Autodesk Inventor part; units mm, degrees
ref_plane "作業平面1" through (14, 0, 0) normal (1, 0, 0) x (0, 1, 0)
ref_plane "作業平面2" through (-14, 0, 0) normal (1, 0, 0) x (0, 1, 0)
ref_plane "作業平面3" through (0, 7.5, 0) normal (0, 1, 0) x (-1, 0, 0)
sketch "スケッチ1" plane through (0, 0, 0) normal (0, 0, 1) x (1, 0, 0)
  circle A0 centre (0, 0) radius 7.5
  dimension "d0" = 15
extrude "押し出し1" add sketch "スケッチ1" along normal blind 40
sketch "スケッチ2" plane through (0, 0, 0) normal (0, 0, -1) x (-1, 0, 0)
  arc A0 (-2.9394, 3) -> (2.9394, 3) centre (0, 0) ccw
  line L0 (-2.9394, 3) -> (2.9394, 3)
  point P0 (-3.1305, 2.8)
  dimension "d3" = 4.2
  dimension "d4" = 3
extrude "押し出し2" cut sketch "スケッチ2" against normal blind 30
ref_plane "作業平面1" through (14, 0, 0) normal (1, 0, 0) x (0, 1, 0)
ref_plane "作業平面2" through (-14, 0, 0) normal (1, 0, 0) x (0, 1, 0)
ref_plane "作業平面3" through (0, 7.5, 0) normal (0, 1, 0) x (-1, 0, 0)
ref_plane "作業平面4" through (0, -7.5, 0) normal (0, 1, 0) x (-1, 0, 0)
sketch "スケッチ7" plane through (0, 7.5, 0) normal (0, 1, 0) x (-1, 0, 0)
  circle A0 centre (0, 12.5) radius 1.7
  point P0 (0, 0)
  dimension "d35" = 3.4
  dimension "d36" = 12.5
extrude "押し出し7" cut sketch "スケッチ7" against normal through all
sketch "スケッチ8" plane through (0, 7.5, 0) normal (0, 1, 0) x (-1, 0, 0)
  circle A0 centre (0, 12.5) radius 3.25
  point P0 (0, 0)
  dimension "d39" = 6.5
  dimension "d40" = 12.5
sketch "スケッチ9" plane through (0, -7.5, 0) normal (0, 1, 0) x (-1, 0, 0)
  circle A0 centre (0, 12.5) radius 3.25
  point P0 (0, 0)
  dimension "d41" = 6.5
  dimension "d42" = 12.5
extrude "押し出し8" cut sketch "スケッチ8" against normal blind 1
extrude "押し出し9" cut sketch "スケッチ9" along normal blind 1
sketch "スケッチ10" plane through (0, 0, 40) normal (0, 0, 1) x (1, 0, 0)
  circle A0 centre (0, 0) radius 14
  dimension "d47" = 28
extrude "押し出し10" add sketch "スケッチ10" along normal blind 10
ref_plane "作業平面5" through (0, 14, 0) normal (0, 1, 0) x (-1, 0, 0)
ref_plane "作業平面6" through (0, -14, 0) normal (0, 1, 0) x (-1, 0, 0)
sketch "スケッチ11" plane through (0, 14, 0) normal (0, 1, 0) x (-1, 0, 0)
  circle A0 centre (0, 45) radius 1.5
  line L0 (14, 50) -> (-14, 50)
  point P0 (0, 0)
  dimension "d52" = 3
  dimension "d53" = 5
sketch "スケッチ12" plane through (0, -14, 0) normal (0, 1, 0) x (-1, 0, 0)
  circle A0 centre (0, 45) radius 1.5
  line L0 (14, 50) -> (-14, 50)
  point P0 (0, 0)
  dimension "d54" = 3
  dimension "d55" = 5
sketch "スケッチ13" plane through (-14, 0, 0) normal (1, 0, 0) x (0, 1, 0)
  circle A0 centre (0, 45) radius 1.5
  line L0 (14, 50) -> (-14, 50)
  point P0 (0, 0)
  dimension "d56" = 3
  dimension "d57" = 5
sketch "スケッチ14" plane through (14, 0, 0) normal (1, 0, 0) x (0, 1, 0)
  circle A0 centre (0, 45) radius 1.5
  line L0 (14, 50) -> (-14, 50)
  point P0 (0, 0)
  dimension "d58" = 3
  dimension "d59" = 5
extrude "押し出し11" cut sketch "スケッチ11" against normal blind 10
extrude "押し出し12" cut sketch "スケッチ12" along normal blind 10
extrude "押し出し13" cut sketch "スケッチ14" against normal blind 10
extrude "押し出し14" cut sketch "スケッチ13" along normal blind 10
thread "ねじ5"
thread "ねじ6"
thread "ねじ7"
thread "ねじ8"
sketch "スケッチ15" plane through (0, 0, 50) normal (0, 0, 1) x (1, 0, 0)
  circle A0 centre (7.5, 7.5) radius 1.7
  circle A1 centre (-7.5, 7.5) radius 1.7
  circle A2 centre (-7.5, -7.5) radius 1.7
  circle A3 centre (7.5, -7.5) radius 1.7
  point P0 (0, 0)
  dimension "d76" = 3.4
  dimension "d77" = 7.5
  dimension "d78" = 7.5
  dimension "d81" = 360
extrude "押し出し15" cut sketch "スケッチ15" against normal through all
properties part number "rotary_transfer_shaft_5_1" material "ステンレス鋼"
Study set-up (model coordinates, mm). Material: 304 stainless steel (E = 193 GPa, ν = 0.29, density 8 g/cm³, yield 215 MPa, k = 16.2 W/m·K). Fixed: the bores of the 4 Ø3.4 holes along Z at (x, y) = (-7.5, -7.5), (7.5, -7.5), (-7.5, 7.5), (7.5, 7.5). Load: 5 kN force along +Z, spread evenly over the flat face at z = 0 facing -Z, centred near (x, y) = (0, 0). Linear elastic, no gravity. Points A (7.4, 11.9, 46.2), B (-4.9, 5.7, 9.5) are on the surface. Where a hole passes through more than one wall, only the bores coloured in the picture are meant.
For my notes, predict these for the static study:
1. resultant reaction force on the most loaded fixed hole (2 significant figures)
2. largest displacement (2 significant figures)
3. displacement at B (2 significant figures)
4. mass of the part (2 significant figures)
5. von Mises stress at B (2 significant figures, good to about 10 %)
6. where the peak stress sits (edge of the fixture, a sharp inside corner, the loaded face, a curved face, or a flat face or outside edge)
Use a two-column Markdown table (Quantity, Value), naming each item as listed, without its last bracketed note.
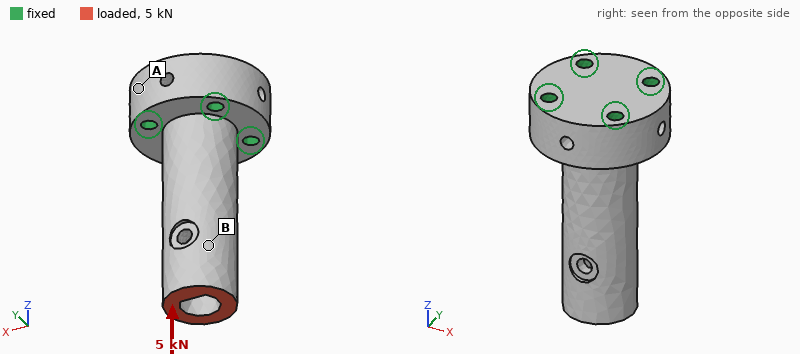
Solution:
| Quantity | Value |
|---|---|
| resultant reaction force on the most loaded fixed hole | 1.3 kN |
| largest displacement | 9.9 µm |
| displacement at B | 7.5 µm |
| mass of the part | 88 g |
| von Mises stress at B | 52 MPa |
| where the peak stress sits | a curved face |
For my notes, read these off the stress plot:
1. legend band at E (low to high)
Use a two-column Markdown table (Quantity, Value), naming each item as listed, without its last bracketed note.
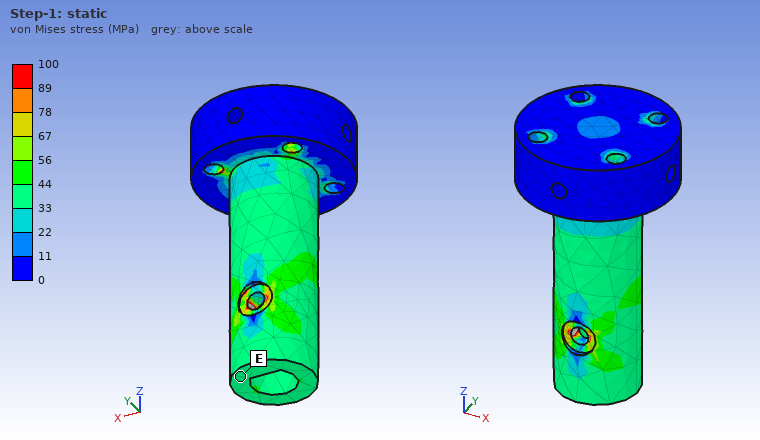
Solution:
| Quantity | Value |
|---|---|
| legend band at E | 33 to 44 MPa |
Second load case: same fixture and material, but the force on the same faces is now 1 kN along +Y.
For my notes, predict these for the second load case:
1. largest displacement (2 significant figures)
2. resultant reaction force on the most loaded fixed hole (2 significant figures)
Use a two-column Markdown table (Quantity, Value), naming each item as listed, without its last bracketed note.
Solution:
| Quantity | Value |
|---|---|
| largest displacement | 70 µm |
| resultant reaction force on the most loaded fixed hole | 1.5 kN |
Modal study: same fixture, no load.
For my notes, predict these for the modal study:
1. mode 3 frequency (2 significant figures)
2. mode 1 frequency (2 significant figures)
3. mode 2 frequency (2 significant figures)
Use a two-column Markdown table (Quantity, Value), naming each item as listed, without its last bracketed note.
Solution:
| Quantity | Value |
|---|---|
| mode 3 frequency | 19 kHz |
| mode 1 frequency | 5900 Hz |
| mode 2 frequency | 5900 Hz |
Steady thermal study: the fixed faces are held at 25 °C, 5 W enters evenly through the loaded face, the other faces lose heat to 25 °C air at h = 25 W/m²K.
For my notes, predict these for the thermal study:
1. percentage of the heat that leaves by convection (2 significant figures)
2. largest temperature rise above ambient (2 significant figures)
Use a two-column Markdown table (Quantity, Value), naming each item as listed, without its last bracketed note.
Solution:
| Quantity | Value |
|---|---|
| percentage of the heat that leaves by convection | 47 % |
| largest temperature rise above ambient | 71 K |
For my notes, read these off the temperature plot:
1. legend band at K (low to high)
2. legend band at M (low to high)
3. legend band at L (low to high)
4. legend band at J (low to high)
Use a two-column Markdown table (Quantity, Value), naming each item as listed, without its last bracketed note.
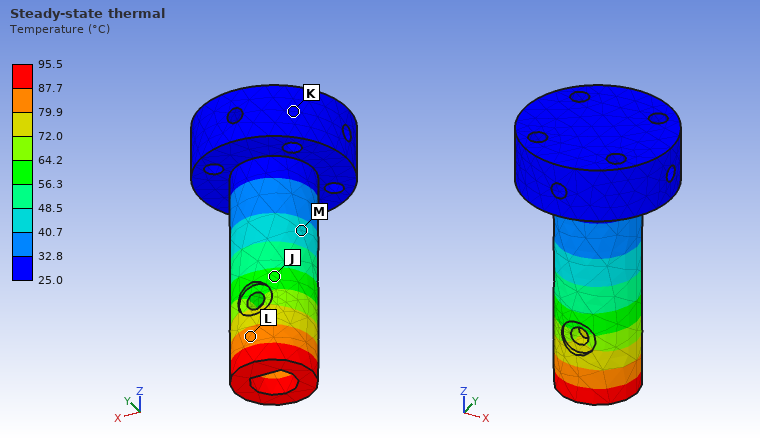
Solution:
| Quantity | Value |
|---|---|
| legend band at K | 25.0 to 32.8 °C |
| legend band at M | 40.7 to 48.5 °C |
| legend band at L | 79.9 to 87.7 °C |
| legend band at J | 56.3 to 64.2 °C |
